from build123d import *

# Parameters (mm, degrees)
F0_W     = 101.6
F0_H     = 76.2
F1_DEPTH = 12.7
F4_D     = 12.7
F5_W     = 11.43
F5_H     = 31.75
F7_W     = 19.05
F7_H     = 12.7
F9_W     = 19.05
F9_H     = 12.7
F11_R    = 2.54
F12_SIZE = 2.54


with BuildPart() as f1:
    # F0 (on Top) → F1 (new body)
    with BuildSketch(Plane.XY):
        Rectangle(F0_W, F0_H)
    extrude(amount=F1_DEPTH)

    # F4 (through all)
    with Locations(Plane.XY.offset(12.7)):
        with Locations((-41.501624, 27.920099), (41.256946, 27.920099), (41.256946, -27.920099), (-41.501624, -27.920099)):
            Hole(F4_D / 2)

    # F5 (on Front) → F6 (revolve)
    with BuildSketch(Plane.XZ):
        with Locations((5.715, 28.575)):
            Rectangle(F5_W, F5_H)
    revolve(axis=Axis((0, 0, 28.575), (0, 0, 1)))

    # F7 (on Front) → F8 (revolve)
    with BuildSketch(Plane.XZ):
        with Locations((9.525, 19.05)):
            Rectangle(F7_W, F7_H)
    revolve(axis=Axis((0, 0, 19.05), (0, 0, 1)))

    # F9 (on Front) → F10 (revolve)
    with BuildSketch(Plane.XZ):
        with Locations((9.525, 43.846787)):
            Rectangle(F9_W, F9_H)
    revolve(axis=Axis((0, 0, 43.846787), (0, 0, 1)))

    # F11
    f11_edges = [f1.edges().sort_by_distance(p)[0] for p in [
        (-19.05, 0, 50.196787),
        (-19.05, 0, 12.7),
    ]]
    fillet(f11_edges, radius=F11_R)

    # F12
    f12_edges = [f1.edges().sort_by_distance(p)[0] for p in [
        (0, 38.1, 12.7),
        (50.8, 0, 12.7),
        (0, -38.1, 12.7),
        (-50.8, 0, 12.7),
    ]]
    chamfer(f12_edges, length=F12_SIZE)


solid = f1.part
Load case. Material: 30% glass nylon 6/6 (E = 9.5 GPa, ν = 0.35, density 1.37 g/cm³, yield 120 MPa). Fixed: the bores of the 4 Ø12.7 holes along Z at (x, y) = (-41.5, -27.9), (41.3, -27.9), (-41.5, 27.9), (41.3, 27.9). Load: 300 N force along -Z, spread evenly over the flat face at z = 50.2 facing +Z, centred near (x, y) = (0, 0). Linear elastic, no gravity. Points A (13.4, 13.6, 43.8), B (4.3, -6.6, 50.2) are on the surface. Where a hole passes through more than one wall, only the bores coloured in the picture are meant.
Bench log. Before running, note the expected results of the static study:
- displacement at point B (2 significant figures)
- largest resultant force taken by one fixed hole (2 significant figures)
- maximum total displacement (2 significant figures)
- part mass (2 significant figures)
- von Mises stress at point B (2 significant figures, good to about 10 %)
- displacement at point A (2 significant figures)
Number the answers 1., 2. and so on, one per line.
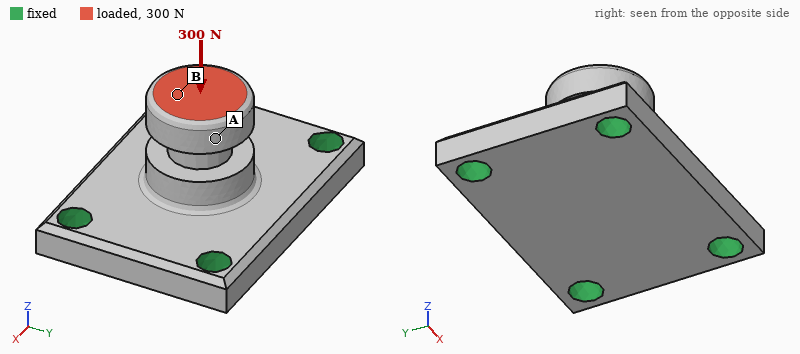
1. 7.7 µm
2. 78 N
3. 7.8 µm
4. 170 g
5. 0.50 MPa
6. 7.7 µm
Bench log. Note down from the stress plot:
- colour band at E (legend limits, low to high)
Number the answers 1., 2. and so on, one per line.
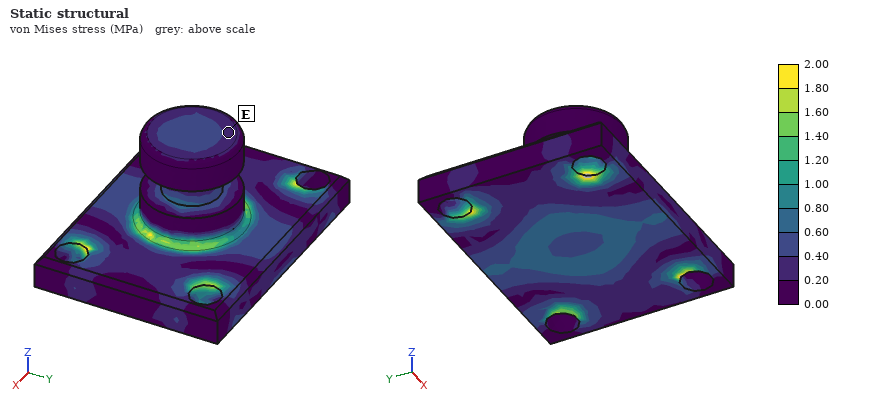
1. 0.20 to 0.40 MPa
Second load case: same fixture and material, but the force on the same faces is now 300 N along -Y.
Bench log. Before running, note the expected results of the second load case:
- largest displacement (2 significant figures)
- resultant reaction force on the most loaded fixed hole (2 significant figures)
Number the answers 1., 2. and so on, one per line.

1. 52 µm
2. 160 N
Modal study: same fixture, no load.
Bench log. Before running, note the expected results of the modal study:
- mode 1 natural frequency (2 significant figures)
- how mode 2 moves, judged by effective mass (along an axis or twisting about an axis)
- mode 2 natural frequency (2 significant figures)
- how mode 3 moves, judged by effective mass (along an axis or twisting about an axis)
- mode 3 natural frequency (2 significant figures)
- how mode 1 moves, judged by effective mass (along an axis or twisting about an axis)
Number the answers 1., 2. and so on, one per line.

1. 3000 Hz
2. along X
3. 3400 Hz
4. along Z
5. 3700 Hz
6. along Y
